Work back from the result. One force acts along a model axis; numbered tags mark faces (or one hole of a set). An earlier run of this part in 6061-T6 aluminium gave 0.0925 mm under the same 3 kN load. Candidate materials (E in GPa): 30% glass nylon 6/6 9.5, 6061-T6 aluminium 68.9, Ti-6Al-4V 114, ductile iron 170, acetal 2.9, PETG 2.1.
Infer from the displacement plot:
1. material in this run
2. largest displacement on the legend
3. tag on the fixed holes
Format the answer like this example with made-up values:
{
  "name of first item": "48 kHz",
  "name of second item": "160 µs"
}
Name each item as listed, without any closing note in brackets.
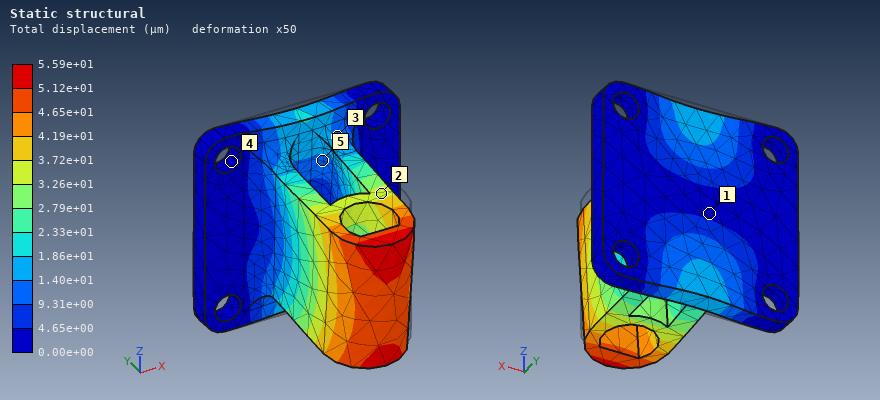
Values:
{
  "material in this run": "Ti-6Al-4V",
  "largest displacement on the legend": "5.59e+01 µm",
  "tag on the fixed holes": "4"
}
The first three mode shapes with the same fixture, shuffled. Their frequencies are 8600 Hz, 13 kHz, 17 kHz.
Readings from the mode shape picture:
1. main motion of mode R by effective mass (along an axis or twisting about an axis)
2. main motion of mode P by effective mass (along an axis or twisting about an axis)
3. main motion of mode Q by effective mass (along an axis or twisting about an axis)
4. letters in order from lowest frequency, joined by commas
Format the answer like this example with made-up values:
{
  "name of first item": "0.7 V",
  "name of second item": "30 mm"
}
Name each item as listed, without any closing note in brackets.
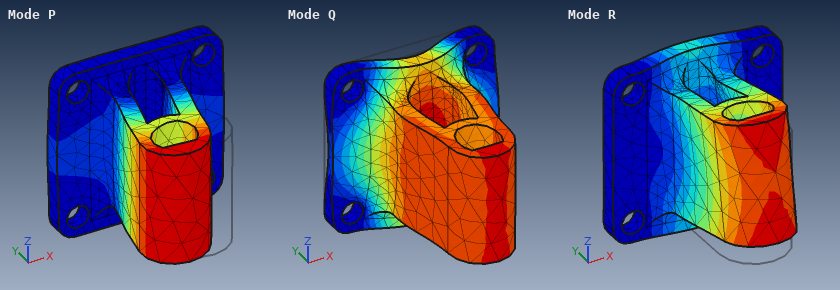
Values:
{
  "main motion of mode R by effective mass": "along Z",
  "main motion of mode P by effective mass": "along X",
  "main motion of mode Q by effective mass": "along Y",
  "letters in order from lowest frequency, joined by commas": "P, R, Q"
}
